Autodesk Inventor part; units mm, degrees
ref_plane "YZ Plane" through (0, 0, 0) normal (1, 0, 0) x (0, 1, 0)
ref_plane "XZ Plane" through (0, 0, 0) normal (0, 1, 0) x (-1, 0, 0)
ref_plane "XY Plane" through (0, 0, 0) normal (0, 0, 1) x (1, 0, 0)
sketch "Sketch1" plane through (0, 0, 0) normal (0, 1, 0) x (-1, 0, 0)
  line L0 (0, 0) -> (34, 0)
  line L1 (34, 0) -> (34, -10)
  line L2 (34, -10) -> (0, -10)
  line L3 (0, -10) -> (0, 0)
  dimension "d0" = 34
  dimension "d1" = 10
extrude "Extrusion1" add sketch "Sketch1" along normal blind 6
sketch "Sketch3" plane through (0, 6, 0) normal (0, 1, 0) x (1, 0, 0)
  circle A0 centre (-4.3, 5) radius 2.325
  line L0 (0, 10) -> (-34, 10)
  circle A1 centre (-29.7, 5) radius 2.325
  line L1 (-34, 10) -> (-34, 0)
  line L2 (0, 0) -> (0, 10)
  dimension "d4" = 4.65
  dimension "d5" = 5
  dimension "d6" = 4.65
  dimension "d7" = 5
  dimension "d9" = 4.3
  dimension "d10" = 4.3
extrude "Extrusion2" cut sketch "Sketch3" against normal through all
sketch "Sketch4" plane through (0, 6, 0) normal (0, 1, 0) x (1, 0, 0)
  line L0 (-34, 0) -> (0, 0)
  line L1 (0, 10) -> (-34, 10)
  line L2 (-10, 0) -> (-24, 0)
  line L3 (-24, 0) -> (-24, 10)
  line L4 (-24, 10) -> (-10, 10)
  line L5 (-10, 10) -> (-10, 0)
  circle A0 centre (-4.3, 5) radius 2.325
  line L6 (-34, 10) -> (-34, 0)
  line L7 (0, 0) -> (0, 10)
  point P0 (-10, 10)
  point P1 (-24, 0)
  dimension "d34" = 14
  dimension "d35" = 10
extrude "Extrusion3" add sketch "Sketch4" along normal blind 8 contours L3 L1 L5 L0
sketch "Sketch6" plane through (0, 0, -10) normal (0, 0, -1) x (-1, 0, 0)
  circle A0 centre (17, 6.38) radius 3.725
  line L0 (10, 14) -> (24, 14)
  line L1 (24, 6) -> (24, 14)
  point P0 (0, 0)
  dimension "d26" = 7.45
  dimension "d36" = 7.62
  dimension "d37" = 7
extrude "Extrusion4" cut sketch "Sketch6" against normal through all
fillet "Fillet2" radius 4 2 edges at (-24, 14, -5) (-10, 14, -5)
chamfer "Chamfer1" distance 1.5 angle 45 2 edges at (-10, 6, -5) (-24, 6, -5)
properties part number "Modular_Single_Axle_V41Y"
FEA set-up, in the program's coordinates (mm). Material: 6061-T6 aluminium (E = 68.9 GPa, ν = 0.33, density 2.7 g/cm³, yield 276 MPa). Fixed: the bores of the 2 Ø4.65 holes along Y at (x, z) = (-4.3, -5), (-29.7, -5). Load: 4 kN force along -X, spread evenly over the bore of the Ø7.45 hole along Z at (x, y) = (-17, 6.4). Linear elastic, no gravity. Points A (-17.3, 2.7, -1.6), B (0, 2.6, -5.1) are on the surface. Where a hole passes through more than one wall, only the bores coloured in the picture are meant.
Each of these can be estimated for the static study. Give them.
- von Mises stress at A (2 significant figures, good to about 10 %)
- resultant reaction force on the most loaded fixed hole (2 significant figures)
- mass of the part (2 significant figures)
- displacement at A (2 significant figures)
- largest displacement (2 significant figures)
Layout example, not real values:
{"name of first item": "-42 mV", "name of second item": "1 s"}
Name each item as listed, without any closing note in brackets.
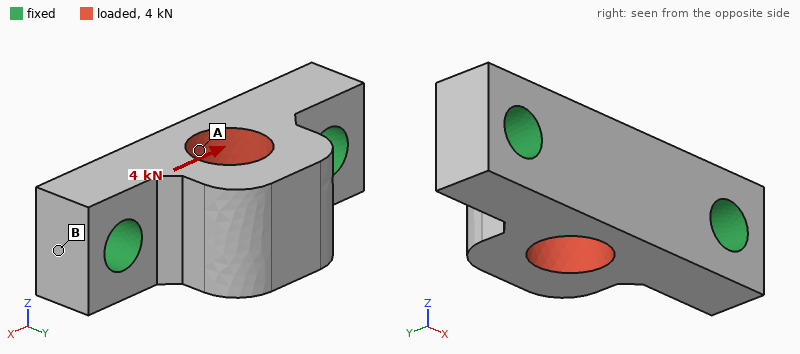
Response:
{"von Mises stress at A": "31 MPa", "resultant reaction force on the most loaded fixed hole": "2.1 kN", "mass of the part": "6.7 g", "displacement at A": "3.2 µm", "largest displacement": "12 µm"}
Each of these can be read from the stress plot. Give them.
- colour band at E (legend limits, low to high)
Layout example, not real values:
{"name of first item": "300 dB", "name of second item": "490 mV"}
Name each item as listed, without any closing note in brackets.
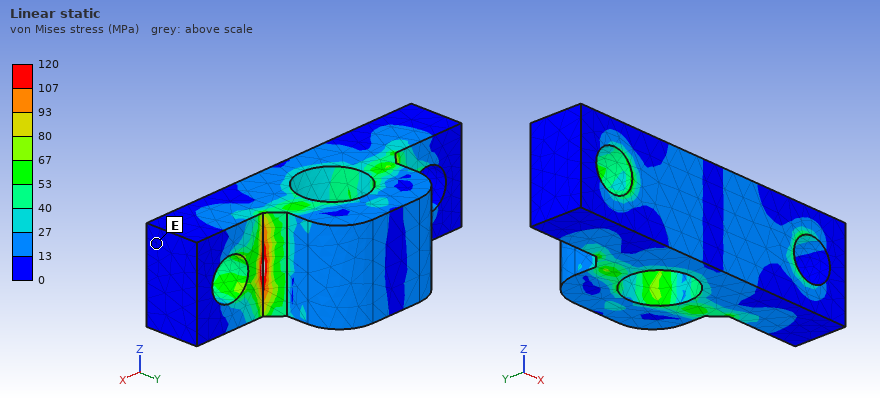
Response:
{"colour band at E": "0 to 13 MPa"}
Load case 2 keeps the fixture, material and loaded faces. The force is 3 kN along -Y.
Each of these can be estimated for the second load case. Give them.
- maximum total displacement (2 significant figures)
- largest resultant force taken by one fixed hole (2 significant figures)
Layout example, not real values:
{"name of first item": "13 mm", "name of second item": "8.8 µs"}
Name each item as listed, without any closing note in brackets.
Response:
{"maximum total displacement": "16 µm", "largest resultant force taken by one fixed hole": "1.5 kN"}
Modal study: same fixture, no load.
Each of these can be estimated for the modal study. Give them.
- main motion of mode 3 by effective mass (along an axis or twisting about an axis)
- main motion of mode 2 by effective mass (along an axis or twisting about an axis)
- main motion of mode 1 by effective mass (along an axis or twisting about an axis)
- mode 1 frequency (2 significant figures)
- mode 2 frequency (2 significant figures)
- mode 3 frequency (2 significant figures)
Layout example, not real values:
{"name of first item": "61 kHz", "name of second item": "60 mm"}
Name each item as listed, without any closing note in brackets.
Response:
{"main motion of mode 3 by effective mass": "along X", "main motion of mode 2 by effective mass": "along Y", "main motion of mode 1 by effective mass": "along Z", "mode 1 frequency": "23 kHz", "mode 2 frequency": "42 kHz", "mode 3 frequency": "48 kHz"}
